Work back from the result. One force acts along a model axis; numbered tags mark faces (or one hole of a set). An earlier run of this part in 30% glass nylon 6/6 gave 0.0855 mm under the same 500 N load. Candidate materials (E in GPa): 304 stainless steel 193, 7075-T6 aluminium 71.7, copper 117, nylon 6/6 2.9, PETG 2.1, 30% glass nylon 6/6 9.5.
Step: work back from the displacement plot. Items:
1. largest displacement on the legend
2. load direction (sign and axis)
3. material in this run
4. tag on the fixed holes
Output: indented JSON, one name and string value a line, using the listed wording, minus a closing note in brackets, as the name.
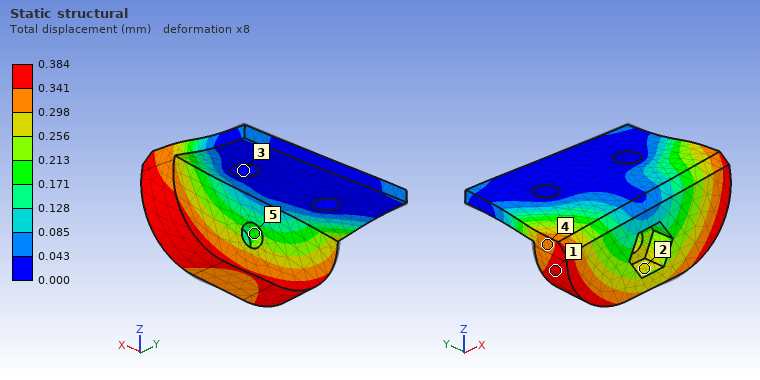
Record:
{
  "largest displacement on the legend": "0.384 mm",
  "load direction": "+X",
  "material in this run": "PETG",
  "tag on the fixed holes": "3"
}
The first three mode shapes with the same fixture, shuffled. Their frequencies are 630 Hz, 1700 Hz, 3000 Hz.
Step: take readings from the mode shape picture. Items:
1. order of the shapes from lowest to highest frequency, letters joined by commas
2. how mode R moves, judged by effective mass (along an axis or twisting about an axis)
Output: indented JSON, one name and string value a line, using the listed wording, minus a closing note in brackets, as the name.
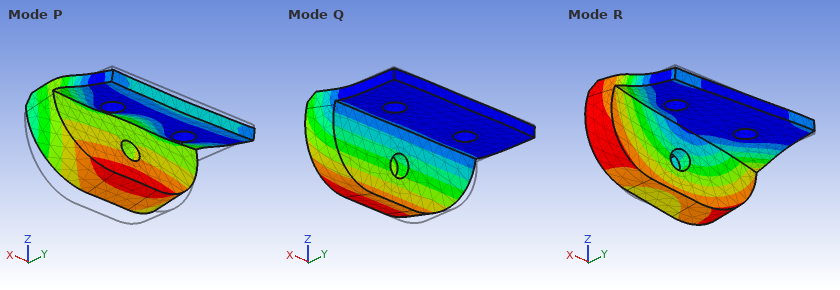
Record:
{
  "order of the shapes from lowest to highest frequency, letters joined by commas": "Q, R, P",
  "how mode R moves, judged by effective mass": "along X"
}
